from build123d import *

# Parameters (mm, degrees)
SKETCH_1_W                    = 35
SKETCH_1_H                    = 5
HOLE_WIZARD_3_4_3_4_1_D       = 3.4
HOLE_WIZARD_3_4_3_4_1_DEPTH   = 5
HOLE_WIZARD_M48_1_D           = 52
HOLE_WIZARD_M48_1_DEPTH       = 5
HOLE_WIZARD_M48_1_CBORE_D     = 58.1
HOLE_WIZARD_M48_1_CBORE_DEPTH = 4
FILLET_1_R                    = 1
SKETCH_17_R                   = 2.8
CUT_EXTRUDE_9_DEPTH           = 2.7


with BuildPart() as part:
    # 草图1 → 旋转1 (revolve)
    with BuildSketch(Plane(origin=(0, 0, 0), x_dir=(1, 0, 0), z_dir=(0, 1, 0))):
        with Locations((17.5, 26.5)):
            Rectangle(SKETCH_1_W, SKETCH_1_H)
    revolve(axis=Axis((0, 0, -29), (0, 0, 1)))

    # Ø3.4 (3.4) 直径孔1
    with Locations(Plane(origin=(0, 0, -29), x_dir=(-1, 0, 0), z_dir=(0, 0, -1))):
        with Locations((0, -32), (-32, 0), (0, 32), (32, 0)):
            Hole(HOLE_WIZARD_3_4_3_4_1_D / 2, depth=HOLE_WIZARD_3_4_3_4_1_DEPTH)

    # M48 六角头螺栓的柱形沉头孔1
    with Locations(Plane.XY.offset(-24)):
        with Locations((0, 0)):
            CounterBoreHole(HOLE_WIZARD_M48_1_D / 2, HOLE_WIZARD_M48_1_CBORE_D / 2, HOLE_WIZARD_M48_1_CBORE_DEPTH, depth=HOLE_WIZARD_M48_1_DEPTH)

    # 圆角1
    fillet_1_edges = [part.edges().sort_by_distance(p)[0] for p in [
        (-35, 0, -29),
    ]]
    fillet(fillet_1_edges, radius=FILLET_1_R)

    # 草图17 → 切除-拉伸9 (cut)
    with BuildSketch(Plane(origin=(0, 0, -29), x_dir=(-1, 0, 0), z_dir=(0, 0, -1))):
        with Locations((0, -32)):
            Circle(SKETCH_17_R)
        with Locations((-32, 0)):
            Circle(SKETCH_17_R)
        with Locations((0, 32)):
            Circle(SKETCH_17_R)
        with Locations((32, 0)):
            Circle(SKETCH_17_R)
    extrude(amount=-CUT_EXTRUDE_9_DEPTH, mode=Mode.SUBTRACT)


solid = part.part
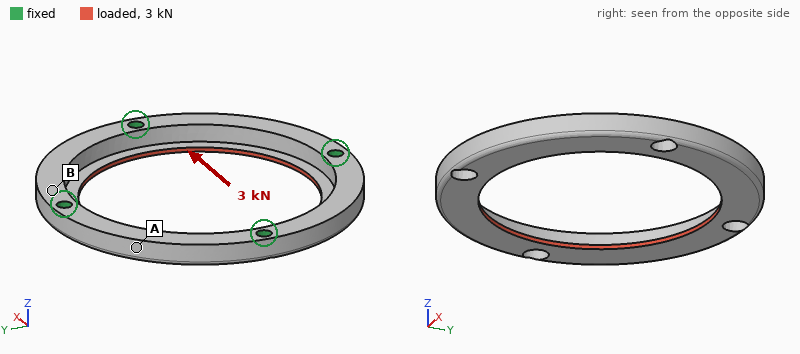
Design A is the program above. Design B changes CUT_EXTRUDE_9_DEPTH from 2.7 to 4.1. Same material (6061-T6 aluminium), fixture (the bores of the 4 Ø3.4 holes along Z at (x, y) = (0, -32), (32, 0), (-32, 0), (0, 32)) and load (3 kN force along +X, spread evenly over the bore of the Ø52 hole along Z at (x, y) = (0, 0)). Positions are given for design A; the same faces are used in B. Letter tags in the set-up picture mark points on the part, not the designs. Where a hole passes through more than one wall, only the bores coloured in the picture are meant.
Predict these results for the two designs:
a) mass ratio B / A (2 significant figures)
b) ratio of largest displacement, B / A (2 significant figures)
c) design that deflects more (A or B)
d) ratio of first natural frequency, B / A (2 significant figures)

0.99
1.8
B
0.71
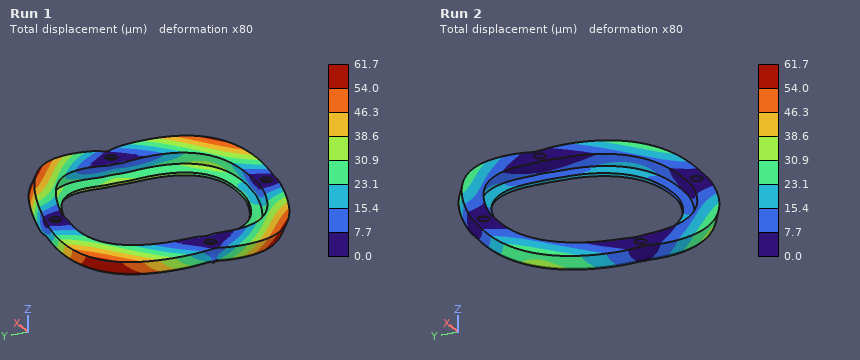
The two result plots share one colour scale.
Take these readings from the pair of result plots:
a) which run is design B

Run 1
